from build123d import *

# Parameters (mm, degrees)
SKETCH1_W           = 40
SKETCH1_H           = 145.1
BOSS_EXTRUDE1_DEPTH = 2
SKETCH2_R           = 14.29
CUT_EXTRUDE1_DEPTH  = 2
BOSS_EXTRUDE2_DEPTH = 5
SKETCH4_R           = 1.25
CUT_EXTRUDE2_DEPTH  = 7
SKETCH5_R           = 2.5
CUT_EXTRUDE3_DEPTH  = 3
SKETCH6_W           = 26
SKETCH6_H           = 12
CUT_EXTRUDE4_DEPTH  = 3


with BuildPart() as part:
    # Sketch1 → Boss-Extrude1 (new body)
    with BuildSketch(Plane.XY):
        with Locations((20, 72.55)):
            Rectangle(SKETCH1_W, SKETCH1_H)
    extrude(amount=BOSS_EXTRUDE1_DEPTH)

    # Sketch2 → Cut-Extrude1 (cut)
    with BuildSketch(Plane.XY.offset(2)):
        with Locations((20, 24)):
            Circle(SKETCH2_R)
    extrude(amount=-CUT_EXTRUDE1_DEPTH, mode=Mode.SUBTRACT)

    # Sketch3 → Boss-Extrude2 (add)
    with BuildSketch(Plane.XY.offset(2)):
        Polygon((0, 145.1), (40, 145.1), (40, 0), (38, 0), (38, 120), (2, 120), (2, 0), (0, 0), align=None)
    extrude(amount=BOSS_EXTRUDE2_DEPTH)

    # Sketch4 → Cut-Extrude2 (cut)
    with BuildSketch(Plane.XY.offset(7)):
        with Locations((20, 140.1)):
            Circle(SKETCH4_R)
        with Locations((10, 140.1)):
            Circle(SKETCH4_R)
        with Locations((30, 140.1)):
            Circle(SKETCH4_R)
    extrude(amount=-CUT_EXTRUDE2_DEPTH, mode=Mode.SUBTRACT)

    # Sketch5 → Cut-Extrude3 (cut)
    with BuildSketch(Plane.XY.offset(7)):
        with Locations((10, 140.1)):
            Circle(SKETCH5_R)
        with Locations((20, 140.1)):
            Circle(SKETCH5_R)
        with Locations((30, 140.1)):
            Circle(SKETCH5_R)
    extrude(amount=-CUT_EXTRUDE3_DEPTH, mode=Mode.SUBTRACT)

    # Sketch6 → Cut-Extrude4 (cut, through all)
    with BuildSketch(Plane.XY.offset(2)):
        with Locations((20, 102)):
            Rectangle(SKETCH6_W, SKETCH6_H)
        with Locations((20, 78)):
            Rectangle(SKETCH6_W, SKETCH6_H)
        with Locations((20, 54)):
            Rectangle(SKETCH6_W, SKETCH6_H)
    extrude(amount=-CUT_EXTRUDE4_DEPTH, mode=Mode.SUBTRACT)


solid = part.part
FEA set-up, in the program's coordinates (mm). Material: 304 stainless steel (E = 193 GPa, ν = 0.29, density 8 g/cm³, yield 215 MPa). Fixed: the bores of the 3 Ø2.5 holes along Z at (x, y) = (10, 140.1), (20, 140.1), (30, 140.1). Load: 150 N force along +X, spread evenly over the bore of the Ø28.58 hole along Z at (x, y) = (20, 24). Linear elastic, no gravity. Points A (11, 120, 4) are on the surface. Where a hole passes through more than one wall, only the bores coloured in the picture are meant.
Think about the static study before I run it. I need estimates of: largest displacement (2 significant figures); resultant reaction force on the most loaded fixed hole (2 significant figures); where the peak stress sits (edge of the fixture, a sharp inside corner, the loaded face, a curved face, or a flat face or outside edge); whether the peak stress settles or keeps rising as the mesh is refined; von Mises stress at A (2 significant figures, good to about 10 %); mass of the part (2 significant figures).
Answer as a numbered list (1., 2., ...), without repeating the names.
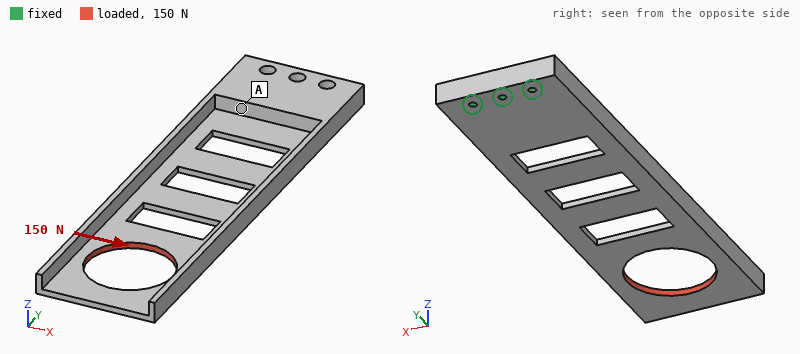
1. 93 µm
2. 810 N
3. edge of the fixture
4. keeps rising
5. 4.7 MPa
6. 130 g
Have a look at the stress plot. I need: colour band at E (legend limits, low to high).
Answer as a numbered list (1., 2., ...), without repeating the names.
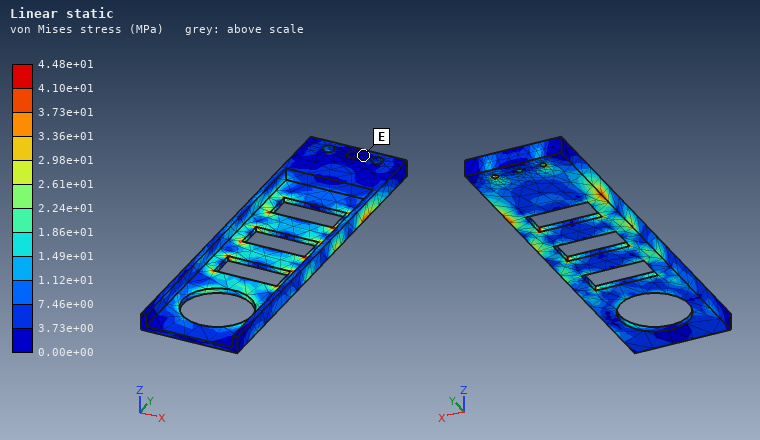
1. 0.00e+00 to 3.73e+00 MPa
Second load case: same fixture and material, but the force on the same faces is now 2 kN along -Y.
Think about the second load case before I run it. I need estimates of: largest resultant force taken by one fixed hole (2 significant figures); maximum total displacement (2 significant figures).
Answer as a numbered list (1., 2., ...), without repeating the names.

1. 770 N
2. 0.56 mm
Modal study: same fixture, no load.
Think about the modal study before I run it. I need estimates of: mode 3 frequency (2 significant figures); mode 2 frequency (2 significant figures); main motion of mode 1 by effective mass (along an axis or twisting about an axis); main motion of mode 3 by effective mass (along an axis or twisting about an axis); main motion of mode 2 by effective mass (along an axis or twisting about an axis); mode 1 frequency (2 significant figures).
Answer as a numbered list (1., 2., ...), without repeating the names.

1. 1500 Hz
2. 630 Hz
3. along Z
4. along X
5. twisting about Y
6. 280 Hz
